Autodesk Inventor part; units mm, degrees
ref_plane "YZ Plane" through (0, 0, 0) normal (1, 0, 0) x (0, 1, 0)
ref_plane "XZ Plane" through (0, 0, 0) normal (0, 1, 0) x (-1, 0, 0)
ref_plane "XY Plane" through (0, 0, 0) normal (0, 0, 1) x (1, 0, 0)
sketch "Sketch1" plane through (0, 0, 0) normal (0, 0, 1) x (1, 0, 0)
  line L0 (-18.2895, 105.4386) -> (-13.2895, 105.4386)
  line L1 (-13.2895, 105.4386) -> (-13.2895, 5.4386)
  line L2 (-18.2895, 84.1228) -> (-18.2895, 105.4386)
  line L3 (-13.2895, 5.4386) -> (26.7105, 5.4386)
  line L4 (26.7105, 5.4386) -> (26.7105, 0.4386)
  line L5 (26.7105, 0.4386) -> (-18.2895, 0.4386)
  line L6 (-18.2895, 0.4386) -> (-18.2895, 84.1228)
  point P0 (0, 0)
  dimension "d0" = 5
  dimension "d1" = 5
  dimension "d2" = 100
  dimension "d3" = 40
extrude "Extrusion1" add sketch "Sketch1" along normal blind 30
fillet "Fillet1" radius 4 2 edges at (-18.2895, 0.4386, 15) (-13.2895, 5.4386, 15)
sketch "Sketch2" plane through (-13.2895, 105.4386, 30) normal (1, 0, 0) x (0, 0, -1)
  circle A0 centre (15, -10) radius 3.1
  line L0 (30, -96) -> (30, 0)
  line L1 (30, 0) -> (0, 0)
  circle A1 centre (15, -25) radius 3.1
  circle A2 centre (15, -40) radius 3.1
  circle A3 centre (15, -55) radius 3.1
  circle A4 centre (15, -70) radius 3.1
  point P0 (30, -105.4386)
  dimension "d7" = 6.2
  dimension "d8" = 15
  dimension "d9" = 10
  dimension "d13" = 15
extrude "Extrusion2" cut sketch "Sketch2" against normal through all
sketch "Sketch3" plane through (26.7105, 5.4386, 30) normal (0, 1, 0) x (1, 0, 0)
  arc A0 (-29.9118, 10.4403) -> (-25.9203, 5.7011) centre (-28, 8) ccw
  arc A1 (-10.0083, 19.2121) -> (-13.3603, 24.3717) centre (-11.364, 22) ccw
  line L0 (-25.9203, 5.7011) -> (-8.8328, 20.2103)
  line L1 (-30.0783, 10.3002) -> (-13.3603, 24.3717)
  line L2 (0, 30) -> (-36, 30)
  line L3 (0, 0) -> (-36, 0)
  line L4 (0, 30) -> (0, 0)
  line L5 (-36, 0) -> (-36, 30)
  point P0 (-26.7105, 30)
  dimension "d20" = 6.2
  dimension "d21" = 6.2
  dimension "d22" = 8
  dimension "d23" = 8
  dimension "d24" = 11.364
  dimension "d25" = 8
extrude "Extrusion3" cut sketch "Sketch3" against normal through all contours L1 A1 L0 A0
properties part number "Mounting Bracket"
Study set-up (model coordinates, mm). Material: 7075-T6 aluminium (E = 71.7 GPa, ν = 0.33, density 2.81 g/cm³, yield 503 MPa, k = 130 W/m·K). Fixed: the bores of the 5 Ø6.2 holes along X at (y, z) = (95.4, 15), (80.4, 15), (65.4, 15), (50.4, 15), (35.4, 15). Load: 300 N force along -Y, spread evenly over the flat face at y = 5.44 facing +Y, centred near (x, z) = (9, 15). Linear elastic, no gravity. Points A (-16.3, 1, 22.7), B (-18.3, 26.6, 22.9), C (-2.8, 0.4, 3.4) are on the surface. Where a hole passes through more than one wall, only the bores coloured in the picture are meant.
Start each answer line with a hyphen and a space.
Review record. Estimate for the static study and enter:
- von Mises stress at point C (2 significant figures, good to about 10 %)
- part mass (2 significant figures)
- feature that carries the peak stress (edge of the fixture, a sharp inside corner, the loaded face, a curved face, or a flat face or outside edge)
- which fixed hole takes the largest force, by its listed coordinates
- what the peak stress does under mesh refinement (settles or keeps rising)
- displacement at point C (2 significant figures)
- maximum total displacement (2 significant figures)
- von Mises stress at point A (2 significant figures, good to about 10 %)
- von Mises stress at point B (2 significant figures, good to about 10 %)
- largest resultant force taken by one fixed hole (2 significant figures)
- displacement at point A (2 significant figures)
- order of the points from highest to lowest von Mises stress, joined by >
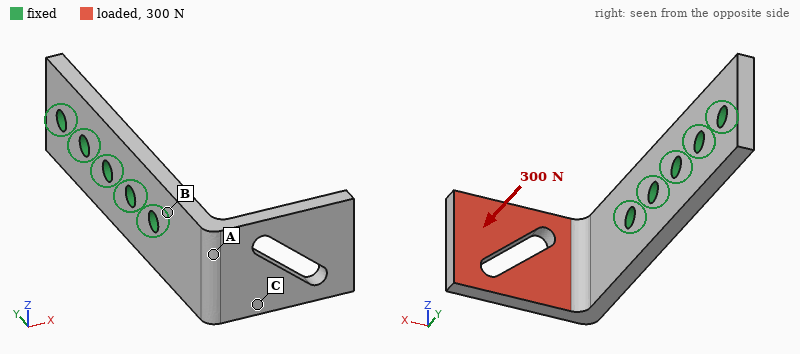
- 34 MPa
- 57 g
- edge of the fixture
- (35.4, 15)
- keeps rising
- 0.23 mm
- 0.61 mm
- 12 MPa
- 53 MPa
- 270 N
- 0.18 mm
- B > C > A
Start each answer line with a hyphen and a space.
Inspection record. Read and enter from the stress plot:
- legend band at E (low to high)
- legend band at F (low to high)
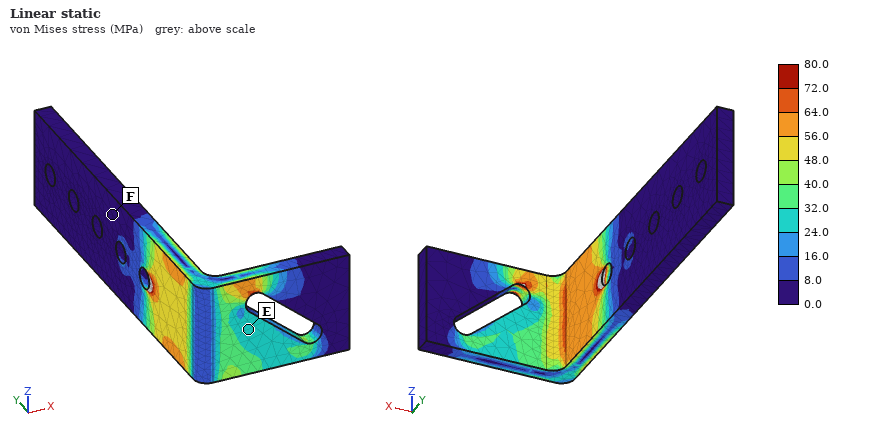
- 24.0 to 32.0 MPa
- 0.0 to 8.0 MPa
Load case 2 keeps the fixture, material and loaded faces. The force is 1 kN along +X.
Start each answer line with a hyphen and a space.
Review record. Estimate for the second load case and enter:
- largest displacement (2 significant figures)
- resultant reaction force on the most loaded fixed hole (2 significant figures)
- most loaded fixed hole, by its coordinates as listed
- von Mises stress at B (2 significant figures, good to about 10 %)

- 0.85 mm
- 1.6 kN
- (35.4, 15)
- 150 MPa
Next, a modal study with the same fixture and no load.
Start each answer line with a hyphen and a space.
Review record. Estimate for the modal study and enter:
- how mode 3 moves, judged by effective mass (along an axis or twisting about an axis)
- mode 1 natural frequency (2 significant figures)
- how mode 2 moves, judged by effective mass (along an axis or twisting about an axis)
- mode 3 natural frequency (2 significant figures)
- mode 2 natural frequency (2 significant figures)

- along X
- 1100 Hz
- along Z
- 2900 Hz
- 1600 Hz
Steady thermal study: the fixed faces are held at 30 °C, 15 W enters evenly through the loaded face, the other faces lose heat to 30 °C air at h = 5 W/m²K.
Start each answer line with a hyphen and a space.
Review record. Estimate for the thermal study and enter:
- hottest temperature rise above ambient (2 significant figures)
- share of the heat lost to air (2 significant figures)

- 52 K
- 3.8 %
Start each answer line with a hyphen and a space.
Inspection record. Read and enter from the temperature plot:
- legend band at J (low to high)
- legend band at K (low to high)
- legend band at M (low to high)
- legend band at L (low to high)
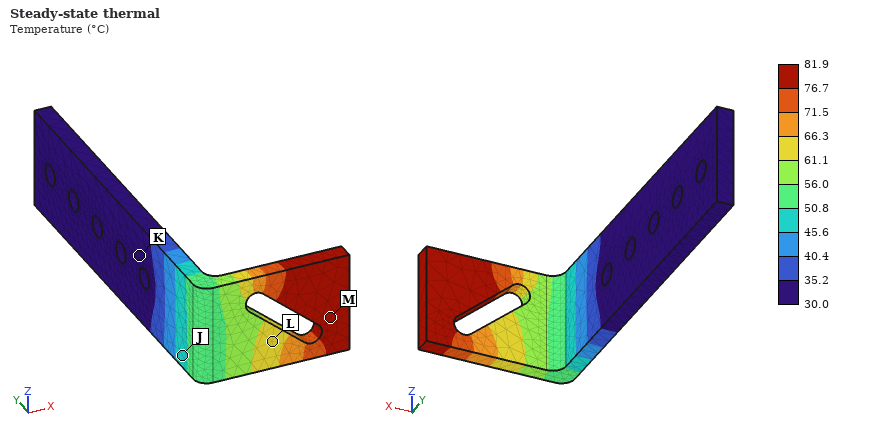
- 45.6 to 50.8 °C
- 30.0 to 35.2 °C
- 76.7 to 81.9 °C
- 61.1 to 66.3 °C
